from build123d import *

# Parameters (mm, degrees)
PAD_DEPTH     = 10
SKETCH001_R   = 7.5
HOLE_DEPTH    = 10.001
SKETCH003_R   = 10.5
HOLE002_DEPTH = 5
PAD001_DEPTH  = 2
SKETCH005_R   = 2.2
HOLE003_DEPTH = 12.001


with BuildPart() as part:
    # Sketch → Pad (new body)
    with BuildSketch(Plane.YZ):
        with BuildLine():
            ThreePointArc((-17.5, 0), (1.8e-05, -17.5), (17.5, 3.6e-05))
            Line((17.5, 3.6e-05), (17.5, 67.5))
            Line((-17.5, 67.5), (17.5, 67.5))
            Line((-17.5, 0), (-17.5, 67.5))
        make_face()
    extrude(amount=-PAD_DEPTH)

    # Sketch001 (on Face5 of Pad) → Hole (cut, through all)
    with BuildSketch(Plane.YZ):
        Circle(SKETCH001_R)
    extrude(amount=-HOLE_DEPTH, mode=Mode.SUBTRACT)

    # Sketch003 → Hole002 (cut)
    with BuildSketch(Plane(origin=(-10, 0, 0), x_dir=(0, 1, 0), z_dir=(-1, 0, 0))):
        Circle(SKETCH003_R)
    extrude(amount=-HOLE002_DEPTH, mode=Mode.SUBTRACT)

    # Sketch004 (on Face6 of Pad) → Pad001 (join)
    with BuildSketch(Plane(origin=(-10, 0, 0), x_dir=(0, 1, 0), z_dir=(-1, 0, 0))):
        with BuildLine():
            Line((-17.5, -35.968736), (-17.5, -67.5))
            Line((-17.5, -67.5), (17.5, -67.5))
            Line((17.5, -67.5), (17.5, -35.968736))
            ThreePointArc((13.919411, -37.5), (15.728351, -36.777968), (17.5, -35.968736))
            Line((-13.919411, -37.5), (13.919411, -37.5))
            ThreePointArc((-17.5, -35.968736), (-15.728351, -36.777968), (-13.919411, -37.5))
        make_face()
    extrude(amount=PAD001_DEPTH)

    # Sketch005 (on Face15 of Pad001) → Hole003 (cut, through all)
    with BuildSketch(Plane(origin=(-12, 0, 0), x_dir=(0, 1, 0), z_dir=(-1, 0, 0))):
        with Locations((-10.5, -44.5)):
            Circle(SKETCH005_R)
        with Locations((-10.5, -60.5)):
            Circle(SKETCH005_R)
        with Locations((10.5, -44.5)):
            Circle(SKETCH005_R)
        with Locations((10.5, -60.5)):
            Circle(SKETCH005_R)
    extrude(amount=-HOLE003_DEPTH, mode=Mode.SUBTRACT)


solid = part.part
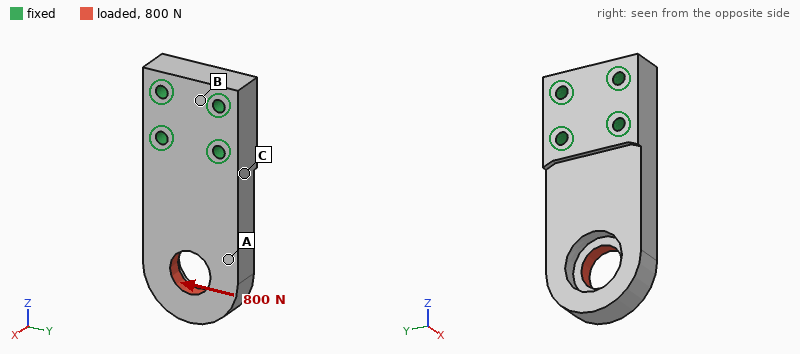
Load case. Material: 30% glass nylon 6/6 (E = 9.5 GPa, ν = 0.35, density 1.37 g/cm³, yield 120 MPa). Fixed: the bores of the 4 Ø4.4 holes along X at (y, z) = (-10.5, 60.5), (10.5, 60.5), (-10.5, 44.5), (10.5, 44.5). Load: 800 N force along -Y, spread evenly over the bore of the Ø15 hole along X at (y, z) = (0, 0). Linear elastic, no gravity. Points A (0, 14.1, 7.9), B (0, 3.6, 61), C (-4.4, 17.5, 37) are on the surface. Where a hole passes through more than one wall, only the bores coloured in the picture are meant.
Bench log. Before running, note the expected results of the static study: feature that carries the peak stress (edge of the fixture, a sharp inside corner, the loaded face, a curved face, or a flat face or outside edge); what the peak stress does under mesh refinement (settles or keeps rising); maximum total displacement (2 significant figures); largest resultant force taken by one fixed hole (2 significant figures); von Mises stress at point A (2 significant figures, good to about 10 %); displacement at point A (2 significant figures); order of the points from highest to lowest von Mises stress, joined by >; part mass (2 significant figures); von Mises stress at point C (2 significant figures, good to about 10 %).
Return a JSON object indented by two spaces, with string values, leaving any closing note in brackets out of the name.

{
  "feature that carries the peak stress": "edge of the fixture",
  "what the peak stress does under mesh refinement": "keeps rising",
  "maximum total displacement": "0.18 mm",
  "largest resultant force taken by one fixed hole": "1.4 kN",
  "von Mises stress at point A": "7.2 MPa",
  "displacement at point A": "0.096 mm",
  "order of the points from highest to lowest von Mises stress, joined by >": "C > A > B",
  "part mass": "37 g",
  "von Mises stress at point C": "11 MPa"
}
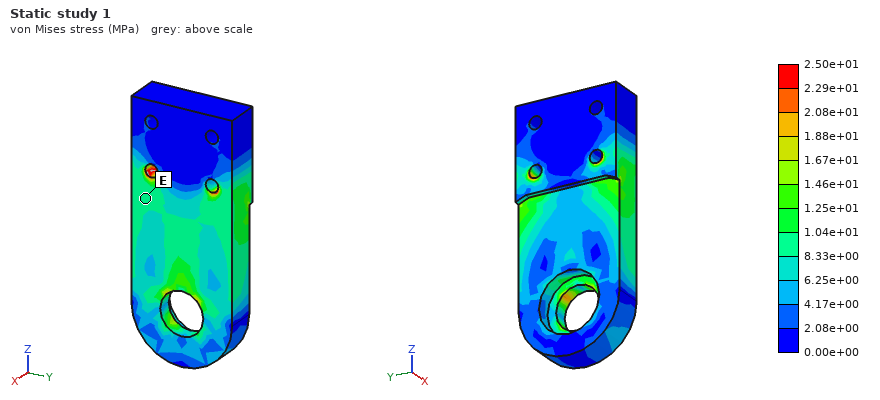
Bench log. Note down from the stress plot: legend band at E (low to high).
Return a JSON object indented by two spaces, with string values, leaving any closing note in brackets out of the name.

{
  "legend band at E": "8.33e+00 to 1.04e+01 MPa"
}
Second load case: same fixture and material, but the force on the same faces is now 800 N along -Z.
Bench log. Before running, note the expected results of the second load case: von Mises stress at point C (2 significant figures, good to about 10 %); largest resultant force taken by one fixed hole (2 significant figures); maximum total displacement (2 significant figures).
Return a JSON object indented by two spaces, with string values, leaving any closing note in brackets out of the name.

{
  "von Mises stress at point C": "2.5 MPa",
  "largest resultant force taken by one fixed hole": "350 N",
  "maximum total displacement": "0.13 mm"
}
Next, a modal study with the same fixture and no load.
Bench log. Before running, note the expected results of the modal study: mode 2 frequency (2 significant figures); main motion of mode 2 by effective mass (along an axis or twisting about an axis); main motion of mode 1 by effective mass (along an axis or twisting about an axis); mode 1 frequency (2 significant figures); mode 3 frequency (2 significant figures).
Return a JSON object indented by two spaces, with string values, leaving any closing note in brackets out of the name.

{
  "mode 2 frequency": "3700 Hz",
  "main motion of mode 2 by effective mass": "along Y",
  "main motion of mode 1 by effective mass": "along X",
  "mode 1 frequency": "1500 Hz",
  "mode 3 frequency": "4100 Hz"
}
